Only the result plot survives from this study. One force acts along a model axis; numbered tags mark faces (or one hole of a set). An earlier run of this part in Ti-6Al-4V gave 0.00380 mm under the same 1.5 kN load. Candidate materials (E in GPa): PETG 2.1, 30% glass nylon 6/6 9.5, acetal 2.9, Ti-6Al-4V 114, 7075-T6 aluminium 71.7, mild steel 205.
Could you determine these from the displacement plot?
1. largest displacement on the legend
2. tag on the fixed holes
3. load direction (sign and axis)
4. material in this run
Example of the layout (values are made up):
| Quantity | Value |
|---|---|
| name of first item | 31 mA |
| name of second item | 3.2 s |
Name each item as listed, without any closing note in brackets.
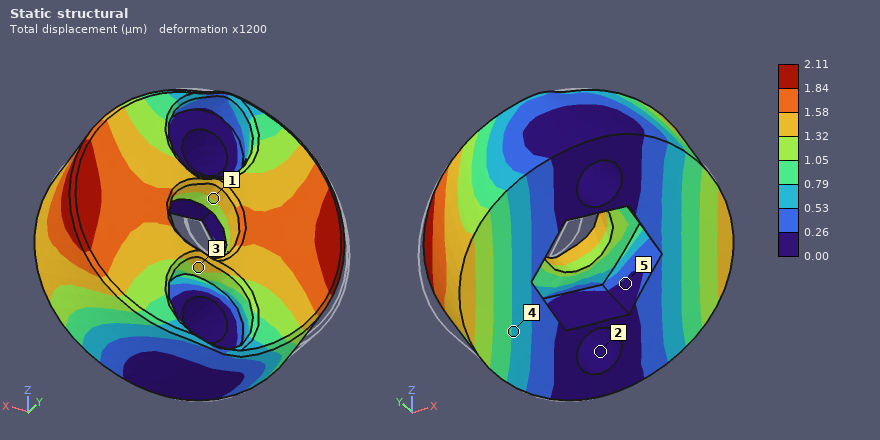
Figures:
| Quantity | Value |
|---|---|
| largest displacement on the legend | 2.11 µm |
| tag on the fixed holes | 2 |
| load direction | +X |
| material in this run | mild steel |
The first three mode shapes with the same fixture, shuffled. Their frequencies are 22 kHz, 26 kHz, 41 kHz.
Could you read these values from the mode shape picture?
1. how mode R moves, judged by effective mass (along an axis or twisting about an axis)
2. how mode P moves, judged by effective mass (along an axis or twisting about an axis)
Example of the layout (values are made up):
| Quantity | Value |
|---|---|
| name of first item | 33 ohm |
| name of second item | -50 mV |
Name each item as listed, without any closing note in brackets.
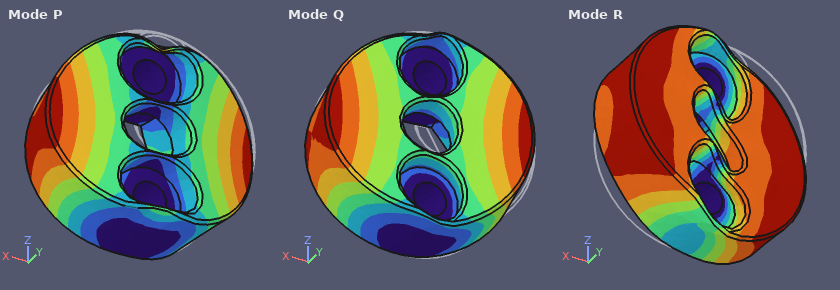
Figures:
| Quantity | Value |
|---|---|
| how mode R moves, judged by effective mass | twisting about Y |
| how mode P moves, judged by effective mass | along Y |
